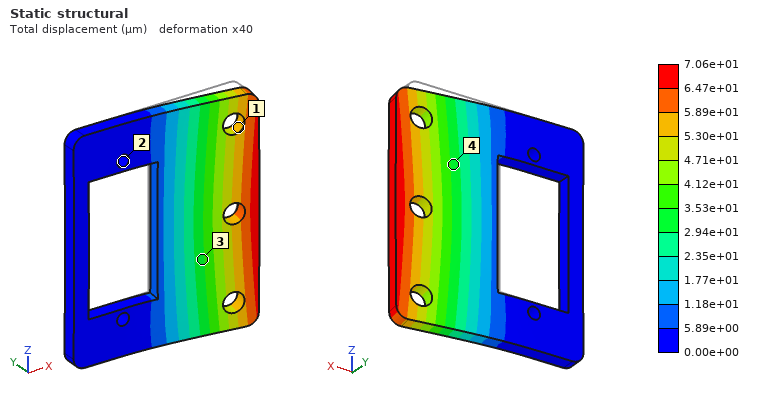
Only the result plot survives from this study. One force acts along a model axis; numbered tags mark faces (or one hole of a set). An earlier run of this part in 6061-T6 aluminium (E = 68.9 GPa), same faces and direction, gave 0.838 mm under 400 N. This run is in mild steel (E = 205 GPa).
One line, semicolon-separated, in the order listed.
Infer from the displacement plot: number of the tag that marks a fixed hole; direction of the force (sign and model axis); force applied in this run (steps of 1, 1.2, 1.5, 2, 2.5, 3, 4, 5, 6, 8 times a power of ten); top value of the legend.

2; -Y; 100 N; 7.06e+01 µm
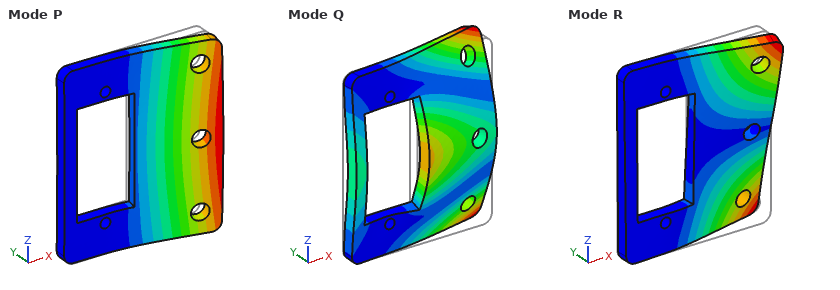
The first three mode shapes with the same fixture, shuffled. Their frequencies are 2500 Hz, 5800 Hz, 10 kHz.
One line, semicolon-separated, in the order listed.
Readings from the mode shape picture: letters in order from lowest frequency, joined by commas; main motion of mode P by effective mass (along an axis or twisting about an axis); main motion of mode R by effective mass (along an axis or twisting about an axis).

P, R, Q; along Y; twisting about X
